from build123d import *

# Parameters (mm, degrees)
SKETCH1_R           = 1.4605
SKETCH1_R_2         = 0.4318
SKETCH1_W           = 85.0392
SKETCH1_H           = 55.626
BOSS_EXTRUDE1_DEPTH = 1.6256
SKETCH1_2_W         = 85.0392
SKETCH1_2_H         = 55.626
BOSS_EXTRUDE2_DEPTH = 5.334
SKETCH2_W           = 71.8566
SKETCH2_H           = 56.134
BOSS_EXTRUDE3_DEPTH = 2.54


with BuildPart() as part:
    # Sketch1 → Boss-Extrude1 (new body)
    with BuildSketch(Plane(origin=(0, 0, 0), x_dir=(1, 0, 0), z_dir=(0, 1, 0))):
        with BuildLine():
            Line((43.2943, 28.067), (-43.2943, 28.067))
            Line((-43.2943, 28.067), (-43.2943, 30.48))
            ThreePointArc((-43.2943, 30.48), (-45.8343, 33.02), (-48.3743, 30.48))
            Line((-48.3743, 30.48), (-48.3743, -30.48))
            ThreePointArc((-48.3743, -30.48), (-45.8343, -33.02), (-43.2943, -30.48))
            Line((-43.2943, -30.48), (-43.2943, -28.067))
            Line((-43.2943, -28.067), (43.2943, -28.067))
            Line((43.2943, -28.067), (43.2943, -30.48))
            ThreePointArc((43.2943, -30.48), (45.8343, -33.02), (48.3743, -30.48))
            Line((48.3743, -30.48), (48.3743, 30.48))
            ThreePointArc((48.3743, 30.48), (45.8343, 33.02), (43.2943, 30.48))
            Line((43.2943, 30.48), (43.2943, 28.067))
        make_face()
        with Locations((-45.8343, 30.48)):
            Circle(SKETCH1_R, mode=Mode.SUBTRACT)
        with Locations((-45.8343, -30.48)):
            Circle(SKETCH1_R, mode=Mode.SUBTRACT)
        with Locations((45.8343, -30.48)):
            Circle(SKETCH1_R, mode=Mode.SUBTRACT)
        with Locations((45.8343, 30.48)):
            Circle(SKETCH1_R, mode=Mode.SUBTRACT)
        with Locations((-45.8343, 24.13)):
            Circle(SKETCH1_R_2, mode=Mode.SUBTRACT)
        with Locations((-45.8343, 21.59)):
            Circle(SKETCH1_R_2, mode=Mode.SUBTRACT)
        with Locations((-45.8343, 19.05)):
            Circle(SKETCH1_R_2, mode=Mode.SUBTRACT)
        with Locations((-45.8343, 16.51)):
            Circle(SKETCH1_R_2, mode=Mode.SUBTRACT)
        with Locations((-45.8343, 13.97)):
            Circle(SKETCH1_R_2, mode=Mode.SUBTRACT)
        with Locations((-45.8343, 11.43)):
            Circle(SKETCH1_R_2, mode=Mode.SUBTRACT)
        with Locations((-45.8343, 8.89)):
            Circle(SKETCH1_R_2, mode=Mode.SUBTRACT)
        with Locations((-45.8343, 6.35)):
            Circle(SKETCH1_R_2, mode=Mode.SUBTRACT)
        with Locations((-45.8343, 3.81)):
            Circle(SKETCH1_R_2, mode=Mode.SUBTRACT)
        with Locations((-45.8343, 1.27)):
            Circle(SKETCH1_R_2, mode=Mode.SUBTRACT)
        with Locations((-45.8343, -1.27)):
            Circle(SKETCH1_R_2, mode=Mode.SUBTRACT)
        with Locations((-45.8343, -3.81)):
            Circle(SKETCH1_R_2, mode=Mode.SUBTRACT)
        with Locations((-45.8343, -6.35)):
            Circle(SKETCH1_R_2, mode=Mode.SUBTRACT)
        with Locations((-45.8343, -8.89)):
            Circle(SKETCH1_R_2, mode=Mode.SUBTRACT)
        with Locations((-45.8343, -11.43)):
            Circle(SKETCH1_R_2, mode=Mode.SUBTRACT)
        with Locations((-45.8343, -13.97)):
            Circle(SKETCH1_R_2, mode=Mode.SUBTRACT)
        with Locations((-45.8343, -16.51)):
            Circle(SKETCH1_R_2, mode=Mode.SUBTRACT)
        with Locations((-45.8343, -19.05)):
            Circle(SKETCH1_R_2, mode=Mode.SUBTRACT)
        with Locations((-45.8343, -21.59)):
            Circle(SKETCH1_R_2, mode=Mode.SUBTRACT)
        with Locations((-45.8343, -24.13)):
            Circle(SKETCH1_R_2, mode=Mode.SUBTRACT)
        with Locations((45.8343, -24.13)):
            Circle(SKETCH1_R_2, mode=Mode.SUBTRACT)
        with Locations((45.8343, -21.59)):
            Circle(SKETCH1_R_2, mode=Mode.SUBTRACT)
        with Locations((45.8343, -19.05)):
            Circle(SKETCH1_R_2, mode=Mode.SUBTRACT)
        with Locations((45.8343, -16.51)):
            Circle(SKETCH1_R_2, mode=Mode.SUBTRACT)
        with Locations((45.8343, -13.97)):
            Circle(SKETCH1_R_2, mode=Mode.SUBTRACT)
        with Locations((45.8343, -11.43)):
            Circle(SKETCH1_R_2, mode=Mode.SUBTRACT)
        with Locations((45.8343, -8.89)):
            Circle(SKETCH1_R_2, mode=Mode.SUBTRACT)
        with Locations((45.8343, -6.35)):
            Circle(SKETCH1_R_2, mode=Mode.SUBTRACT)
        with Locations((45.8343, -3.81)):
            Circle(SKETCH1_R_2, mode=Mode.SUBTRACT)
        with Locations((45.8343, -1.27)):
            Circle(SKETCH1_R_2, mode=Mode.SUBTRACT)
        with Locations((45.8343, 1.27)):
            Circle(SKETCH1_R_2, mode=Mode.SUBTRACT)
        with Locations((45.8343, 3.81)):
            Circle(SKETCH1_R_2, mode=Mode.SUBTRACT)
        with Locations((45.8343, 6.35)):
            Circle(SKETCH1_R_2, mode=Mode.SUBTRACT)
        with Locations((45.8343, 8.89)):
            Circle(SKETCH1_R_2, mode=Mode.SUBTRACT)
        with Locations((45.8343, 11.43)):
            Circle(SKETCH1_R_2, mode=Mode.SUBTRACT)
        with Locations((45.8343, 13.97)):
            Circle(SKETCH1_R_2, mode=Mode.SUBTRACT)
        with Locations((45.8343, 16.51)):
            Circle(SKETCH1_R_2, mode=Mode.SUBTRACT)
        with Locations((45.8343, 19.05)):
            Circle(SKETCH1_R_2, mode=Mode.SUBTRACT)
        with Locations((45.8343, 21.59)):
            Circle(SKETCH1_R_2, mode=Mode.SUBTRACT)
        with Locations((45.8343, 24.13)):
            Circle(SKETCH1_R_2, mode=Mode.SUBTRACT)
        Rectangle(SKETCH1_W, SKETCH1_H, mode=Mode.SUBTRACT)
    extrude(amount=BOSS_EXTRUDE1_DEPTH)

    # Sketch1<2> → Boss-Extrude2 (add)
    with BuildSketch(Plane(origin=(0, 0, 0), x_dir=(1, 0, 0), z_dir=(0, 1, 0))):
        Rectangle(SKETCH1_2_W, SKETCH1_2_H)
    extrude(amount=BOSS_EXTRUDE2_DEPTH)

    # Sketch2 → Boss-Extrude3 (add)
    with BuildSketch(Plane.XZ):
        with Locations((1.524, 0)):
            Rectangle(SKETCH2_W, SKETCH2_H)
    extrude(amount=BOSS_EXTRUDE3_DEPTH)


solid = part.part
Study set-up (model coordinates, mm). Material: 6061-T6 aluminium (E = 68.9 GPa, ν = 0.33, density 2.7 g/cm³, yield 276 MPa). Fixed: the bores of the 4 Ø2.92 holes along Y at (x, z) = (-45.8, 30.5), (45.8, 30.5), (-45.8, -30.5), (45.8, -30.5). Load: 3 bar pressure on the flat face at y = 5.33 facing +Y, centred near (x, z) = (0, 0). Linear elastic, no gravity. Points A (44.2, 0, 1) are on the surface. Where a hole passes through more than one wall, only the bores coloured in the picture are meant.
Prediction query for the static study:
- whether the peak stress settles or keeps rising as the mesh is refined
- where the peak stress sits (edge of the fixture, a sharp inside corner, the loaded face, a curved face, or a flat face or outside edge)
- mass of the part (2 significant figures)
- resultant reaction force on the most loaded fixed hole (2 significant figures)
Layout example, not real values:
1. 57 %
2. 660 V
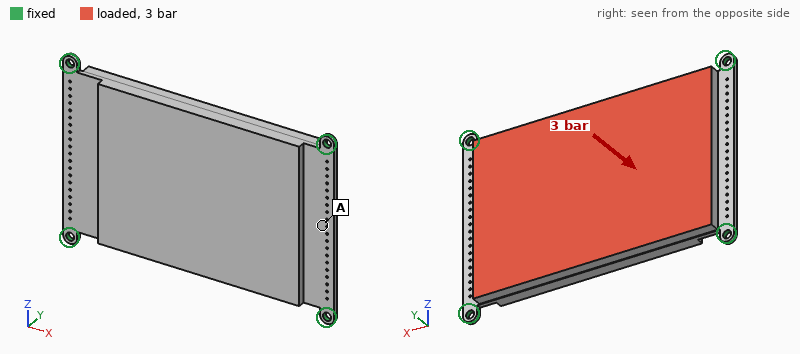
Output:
1. keeps rising
2. edge of the fixture
3. 99 g
4. 470 N
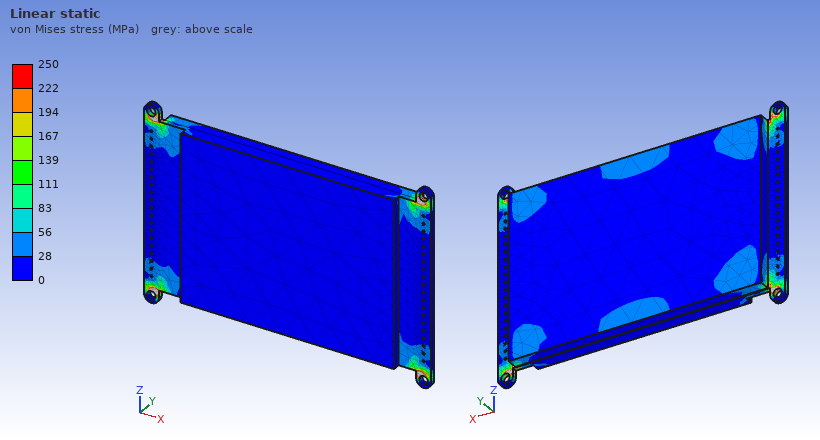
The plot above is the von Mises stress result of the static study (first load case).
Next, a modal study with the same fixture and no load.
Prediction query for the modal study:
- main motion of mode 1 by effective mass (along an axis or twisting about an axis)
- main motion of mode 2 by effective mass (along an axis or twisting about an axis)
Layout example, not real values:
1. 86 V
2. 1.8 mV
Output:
1. along Y
2. twisting about X
